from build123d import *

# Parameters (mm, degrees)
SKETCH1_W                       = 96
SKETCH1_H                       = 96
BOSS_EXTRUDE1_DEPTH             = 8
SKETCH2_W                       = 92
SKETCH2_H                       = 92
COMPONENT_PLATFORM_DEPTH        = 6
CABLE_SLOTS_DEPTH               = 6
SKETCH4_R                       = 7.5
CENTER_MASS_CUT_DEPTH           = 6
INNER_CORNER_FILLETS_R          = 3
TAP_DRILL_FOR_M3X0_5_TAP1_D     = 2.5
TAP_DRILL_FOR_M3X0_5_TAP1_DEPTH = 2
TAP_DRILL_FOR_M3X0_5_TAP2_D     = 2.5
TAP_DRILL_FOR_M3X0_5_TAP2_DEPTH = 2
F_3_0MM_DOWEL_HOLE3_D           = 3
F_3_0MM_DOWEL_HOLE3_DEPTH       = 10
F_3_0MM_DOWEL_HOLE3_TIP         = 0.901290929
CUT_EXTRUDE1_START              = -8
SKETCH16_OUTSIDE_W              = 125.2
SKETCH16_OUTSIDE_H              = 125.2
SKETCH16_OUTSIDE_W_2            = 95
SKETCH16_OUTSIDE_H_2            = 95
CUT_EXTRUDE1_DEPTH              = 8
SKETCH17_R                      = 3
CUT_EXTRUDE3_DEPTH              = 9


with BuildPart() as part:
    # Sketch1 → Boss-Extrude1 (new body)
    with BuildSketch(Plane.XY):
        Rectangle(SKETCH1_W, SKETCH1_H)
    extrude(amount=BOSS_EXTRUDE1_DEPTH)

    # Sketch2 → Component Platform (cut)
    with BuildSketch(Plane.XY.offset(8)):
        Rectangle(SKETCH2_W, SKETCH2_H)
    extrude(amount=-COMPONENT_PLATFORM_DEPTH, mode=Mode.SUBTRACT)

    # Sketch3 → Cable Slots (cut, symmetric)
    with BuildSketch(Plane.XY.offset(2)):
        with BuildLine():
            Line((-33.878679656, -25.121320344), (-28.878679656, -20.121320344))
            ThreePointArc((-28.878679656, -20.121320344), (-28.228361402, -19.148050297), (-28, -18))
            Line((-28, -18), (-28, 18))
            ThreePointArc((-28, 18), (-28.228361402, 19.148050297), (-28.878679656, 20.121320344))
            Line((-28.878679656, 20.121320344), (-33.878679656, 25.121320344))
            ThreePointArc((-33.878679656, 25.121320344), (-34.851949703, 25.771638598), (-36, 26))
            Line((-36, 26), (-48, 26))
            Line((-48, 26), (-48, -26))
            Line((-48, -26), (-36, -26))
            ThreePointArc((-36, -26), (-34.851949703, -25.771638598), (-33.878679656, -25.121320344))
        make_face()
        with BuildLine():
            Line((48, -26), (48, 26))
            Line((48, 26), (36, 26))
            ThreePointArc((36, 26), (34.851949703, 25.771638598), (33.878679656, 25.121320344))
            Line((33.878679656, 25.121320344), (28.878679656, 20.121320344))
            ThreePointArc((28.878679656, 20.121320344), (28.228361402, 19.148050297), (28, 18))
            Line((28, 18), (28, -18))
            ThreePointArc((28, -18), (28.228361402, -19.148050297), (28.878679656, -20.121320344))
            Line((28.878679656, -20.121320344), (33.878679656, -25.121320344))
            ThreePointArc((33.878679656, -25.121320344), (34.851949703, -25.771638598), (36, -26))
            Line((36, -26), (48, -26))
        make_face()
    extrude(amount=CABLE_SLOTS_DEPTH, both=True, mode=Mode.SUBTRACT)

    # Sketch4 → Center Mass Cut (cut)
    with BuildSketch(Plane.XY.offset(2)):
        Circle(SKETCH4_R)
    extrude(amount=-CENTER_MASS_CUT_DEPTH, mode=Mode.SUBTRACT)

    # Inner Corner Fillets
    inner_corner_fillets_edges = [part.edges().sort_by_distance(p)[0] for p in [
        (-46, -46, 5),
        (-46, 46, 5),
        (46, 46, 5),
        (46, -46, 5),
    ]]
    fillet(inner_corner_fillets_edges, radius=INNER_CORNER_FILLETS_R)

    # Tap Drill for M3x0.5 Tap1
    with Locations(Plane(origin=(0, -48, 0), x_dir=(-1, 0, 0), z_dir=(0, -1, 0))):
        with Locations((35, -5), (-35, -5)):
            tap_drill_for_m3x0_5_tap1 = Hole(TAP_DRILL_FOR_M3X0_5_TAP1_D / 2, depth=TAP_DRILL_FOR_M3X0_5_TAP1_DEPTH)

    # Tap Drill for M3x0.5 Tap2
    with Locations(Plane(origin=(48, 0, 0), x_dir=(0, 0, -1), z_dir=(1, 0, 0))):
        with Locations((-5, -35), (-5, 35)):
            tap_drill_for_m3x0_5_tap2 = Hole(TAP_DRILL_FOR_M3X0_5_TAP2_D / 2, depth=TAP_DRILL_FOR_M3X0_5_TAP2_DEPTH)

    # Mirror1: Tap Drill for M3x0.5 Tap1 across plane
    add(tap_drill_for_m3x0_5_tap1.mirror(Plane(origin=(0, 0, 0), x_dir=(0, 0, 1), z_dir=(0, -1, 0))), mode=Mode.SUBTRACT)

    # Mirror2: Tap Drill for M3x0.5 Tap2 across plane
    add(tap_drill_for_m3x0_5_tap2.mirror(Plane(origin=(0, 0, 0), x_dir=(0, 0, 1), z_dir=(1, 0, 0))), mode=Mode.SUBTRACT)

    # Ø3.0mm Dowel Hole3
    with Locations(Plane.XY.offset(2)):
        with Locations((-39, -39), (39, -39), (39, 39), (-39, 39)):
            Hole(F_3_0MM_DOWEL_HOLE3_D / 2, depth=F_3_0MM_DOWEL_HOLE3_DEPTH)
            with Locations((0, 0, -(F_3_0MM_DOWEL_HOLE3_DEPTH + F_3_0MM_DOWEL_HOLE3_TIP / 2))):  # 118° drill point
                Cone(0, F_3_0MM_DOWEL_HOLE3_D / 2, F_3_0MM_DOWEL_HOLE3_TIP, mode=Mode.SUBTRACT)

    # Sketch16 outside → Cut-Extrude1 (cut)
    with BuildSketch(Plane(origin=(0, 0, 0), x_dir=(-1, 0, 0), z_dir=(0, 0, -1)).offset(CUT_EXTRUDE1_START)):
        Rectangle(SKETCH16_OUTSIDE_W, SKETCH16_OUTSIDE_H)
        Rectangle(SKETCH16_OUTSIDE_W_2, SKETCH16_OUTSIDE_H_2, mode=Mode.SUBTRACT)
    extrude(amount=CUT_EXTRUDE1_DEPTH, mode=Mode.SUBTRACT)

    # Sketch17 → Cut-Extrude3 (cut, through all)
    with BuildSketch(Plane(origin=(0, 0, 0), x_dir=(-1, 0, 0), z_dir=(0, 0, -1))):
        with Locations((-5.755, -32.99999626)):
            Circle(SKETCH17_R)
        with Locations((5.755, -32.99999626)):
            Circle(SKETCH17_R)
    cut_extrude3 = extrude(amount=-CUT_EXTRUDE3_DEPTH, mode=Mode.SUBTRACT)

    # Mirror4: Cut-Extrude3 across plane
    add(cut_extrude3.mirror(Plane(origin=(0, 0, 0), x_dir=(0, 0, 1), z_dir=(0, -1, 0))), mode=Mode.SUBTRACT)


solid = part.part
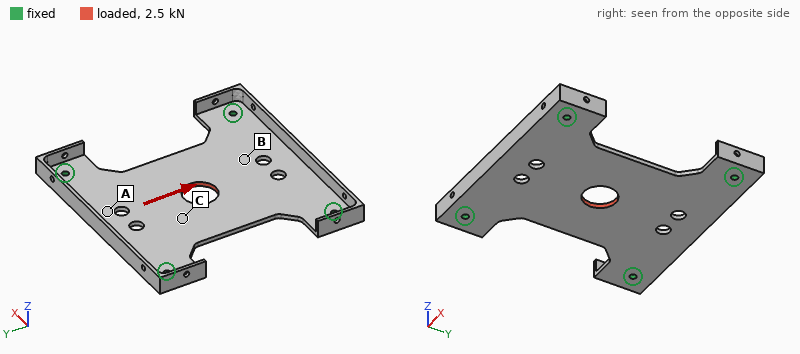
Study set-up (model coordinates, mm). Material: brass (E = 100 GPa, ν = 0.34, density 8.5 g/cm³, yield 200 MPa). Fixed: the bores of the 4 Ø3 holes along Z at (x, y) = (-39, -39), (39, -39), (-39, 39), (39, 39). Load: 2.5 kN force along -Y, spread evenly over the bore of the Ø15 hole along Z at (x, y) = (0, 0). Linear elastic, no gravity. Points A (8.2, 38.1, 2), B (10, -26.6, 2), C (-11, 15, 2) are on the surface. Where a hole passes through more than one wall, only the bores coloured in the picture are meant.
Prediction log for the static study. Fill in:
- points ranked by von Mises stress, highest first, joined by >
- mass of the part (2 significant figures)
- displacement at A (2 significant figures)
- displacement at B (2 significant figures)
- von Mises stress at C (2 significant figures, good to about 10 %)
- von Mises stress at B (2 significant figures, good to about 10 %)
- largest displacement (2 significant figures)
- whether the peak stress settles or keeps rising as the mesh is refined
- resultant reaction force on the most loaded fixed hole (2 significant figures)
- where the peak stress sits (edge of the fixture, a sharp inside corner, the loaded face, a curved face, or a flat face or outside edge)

C > B > A
140 g
16 µm
14 µm
20 MPa
12 MPa
21 µm
keeps rising
720 N
edge of the fixture
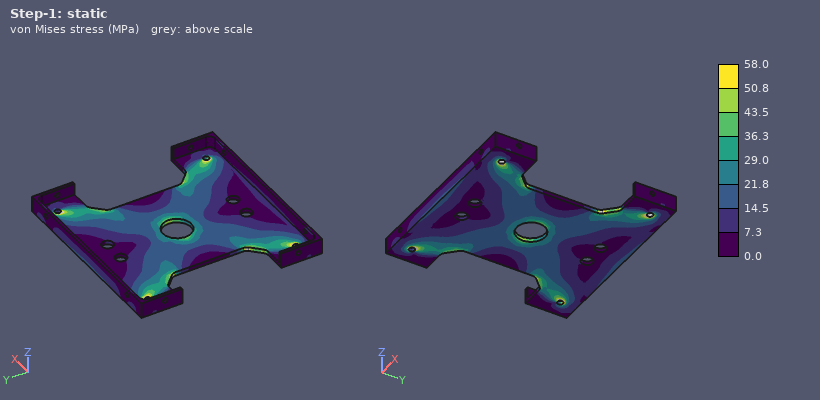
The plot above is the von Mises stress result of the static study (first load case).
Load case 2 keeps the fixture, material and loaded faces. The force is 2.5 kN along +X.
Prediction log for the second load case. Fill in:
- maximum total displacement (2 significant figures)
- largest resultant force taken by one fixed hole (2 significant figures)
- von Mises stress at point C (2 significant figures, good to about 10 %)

15 µm
740 N
22 MPa
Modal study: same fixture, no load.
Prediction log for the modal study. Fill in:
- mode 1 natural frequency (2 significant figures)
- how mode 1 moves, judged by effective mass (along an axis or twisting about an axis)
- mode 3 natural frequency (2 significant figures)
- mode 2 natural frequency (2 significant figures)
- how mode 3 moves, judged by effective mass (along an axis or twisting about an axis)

790 Hz
along Z
1700 Hz
1600 Hz
twisting about X
